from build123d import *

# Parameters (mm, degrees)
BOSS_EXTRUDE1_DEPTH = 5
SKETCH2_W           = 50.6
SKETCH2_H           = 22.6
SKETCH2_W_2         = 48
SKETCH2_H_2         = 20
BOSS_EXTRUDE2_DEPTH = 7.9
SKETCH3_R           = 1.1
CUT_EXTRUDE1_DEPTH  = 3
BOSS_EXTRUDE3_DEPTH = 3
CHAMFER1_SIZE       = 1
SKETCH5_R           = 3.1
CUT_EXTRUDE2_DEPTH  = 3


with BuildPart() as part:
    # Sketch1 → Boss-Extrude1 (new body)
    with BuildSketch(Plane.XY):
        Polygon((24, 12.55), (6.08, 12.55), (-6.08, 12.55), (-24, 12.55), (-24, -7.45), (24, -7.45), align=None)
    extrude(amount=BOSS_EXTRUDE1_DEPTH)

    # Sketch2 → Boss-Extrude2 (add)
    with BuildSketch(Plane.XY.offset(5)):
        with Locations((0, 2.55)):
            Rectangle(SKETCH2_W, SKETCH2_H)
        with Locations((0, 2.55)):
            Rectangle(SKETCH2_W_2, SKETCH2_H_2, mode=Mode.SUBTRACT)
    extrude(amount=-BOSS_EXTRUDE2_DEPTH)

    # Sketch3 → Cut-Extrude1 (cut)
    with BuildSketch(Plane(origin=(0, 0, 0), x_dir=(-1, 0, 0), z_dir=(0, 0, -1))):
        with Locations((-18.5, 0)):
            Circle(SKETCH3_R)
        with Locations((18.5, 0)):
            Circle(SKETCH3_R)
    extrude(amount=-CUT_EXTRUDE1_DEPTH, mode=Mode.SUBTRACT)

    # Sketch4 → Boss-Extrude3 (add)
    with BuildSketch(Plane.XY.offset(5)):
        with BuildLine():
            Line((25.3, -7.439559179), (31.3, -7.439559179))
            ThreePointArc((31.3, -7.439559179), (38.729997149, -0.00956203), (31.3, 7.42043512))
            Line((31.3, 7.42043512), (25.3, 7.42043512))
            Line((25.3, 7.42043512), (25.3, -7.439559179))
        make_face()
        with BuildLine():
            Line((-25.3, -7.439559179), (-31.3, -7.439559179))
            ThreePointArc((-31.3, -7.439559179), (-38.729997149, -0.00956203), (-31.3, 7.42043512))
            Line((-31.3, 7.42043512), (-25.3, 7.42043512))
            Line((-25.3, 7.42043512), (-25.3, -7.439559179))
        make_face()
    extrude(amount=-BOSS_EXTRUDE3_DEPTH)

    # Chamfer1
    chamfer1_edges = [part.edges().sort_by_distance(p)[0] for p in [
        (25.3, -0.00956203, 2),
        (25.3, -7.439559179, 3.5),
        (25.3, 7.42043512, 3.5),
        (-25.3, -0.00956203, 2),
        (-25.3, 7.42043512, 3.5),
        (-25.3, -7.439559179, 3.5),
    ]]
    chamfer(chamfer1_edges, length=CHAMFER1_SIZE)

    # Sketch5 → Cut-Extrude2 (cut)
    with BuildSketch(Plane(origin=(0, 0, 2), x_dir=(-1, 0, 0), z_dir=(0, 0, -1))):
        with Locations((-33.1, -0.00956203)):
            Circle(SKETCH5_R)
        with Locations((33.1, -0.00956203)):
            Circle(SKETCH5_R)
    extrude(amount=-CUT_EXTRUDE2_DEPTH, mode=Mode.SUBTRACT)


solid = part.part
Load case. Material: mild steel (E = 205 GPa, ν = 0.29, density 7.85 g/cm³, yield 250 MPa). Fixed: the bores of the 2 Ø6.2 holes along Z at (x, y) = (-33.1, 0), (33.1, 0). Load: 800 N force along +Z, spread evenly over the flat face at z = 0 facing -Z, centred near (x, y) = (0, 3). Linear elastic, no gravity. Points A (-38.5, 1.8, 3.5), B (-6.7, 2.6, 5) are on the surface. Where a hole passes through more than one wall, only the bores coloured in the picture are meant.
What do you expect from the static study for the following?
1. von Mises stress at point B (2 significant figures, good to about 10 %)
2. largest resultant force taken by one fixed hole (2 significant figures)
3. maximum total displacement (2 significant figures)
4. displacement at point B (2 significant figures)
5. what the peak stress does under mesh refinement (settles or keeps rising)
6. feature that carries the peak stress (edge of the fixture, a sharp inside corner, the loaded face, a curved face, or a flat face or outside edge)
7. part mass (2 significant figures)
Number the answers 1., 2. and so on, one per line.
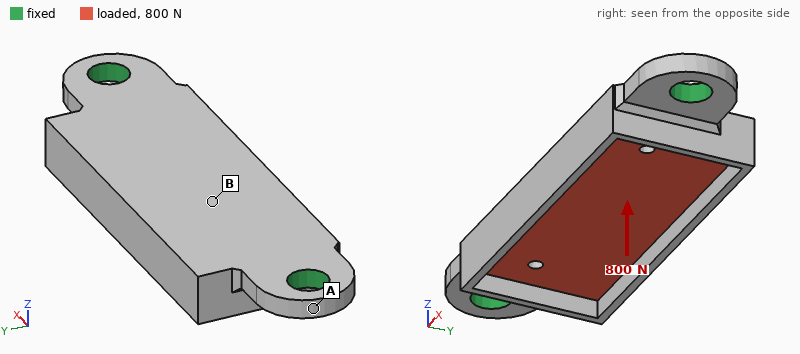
1. 26 MPa
2. 730 N
3. 30 µm
4. 22 µm
5. keeps rising
6. edge of the fixture
7. 56 g
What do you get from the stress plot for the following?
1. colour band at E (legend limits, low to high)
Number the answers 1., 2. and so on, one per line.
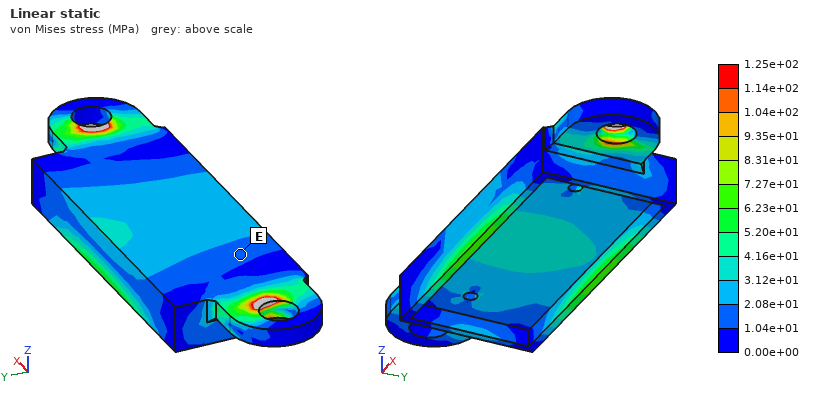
1. 1.04e+01 to 2.08e+01 MPa
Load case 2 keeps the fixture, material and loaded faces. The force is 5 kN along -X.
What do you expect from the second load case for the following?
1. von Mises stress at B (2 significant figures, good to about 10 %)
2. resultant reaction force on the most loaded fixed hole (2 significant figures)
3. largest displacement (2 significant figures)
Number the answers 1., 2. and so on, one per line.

1. 9.5 MPa
2. 2.5 kN
3. 4.8 µm
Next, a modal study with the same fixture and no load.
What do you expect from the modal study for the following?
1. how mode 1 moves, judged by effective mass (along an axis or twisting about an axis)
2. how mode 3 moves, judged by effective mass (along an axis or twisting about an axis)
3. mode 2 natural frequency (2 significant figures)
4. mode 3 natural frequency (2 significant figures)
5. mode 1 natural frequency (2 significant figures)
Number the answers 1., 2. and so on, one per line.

1. along Z
2. twisting about Y
3. 6500 Hz
4. 12 kHz
5. 4600 Hz
